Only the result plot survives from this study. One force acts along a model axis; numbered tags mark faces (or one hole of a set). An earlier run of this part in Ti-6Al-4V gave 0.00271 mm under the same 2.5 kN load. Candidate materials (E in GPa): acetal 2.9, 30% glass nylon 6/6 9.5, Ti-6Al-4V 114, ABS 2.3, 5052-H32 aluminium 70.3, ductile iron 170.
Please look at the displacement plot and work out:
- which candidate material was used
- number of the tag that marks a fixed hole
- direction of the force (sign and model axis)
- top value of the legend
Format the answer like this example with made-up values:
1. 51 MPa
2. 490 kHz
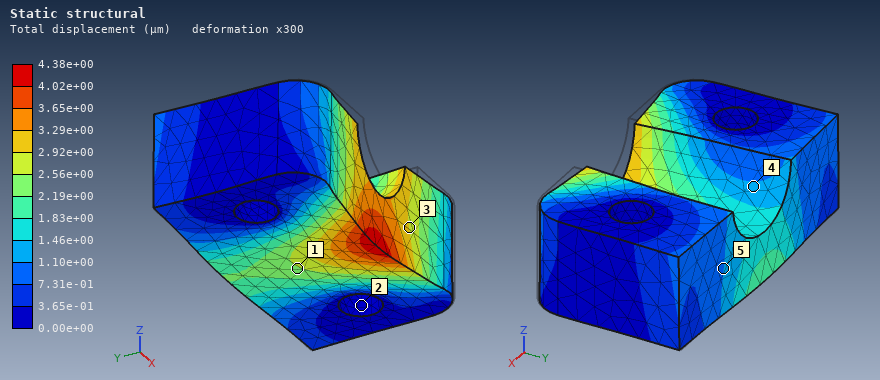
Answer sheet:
1. 5052-H32 aluminium
2. 2
3. +Y
4. 4.38e+00 µm
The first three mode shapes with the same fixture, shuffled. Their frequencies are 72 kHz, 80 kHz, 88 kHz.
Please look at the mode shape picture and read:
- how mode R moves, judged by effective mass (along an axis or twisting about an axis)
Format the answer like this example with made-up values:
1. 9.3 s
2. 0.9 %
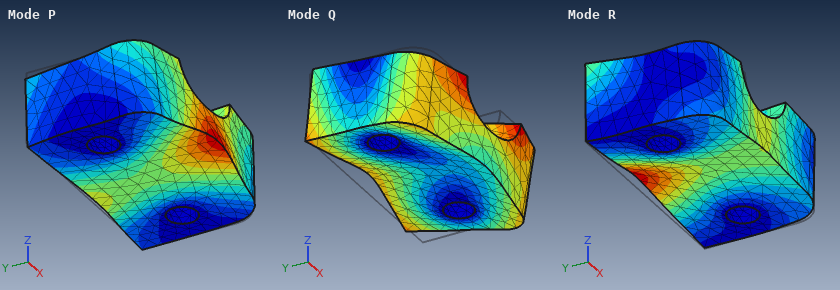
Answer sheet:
1. along Z
